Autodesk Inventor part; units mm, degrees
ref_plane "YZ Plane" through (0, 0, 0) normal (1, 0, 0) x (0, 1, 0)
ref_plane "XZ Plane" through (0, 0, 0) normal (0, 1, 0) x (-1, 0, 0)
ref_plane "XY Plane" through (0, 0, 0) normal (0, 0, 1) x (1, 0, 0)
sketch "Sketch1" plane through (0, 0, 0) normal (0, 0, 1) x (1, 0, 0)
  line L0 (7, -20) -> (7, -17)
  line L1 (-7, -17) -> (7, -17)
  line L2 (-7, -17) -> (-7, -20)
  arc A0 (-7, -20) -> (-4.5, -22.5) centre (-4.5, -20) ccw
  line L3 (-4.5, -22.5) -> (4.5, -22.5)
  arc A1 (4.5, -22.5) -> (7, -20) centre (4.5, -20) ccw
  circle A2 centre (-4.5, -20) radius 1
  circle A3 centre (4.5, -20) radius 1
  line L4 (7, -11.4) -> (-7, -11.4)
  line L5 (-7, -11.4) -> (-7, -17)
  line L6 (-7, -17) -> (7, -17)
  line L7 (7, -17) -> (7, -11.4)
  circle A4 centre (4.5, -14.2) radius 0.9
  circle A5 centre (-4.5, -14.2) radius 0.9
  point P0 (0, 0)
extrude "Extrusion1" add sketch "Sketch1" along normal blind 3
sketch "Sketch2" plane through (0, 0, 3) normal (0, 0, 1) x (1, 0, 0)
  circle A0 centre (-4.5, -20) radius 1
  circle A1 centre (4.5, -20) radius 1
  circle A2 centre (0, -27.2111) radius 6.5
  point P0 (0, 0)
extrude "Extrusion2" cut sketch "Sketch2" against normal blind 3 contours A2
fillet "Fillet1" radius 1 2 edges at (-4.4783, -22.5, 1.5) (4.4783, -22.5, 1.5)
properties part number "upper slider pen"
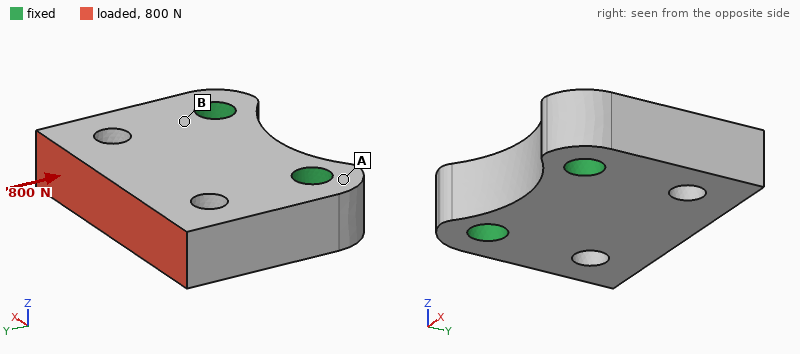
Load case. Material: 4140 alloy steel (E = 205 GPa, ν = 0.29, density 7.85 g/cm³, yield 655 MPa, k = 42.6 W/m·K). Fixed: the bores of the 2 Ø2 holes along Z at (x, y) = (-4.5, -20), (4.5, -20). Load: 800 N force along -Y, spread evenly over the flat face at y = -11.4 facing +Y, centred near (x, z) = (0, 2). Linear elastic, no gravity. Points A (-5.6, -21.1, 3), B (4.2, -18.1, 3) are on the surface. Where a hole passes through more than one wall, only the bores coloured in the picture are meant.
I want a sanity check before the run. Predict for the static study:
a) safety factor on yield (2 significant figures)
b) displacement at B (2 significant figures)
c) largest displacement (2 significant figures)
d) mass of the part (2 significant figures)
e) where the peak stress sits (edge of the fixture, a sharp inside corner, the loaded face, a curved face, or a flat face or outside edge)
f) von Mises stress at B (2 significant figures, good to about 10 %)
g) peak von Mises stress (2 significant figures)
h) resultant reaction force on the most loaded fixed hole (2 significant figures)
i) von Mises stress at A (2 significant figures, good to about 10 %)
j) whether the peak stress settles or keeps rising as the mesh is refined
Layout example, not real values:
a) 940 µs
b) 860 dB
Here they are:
a) 9.1
b) 0.17 µm
c) 1.1 µm
d) 3.1 g
e) a curved face
f) 30 MPa
g) 72 MPa
h) 410 N
i) 8.5 MPa
j) settles
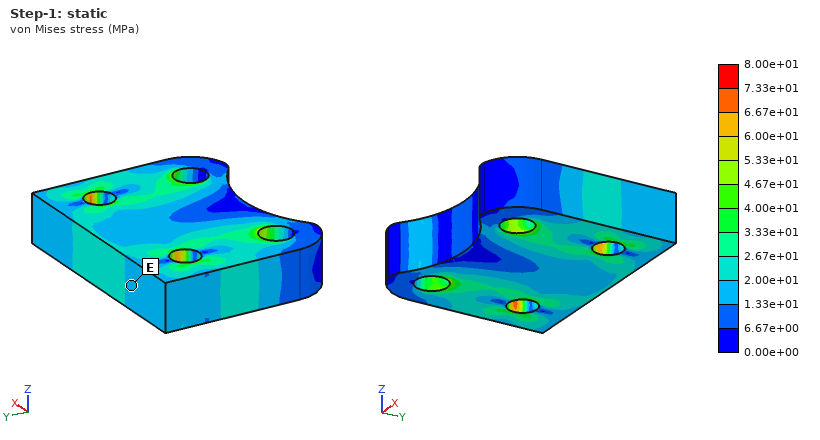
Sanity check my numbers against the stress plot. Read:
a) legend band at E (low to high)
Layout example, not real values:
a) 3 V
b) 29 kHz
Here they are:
a) 1.33e+01 to 2.00e+01 MPa
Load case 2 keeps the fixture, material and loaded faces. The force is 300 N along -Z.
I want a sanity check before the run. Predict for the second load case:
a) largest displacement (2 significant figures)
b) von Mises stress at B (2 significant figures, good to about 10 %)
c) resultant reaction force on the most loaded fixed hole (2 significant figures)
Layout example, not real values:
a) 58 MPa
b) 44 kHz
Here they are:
a) 12 µm
b) 140 MPa
c) 150 N
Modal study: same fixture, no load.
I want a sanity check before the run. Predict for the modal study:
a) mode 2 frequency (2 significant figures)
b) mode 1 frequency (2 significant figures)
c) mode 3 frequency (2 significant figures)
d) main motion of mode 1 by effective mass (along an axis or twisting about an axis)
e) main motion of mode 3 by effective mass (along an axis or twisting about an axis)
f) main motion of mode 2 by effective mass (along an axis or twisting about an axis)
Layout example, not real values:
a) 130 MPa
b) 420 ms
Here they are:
a) 51 kHz
b) 31 kHz
c) 73 kHz
d) along Z
e) along X
f) twisting about Y
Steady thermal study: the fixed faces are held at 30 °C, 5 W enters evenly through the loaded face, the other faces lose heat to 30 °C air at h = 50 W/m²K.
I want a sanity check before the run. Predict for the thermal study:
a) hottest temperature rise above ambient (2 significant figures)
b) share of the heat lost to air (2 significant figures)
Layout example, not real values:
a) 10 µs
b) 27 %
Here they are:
a) 26 K
b) 4.2 %
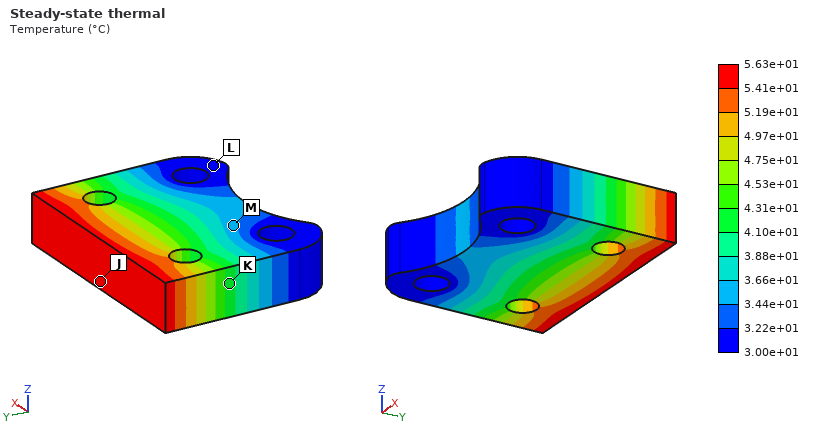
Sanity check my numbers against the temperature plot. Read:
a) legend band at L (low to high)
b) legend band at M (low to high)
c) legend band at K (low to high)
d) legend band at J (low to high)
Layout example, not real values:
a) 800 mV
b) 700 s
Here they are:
a) 3.00e+01 to 3.22e+01 °C
b) 3.44e+01 to 3.66e+01 °C
c) 4.10e+01 to 4.31e+01 °C
d) 5.41e+01 to 5.63e+01 °C
